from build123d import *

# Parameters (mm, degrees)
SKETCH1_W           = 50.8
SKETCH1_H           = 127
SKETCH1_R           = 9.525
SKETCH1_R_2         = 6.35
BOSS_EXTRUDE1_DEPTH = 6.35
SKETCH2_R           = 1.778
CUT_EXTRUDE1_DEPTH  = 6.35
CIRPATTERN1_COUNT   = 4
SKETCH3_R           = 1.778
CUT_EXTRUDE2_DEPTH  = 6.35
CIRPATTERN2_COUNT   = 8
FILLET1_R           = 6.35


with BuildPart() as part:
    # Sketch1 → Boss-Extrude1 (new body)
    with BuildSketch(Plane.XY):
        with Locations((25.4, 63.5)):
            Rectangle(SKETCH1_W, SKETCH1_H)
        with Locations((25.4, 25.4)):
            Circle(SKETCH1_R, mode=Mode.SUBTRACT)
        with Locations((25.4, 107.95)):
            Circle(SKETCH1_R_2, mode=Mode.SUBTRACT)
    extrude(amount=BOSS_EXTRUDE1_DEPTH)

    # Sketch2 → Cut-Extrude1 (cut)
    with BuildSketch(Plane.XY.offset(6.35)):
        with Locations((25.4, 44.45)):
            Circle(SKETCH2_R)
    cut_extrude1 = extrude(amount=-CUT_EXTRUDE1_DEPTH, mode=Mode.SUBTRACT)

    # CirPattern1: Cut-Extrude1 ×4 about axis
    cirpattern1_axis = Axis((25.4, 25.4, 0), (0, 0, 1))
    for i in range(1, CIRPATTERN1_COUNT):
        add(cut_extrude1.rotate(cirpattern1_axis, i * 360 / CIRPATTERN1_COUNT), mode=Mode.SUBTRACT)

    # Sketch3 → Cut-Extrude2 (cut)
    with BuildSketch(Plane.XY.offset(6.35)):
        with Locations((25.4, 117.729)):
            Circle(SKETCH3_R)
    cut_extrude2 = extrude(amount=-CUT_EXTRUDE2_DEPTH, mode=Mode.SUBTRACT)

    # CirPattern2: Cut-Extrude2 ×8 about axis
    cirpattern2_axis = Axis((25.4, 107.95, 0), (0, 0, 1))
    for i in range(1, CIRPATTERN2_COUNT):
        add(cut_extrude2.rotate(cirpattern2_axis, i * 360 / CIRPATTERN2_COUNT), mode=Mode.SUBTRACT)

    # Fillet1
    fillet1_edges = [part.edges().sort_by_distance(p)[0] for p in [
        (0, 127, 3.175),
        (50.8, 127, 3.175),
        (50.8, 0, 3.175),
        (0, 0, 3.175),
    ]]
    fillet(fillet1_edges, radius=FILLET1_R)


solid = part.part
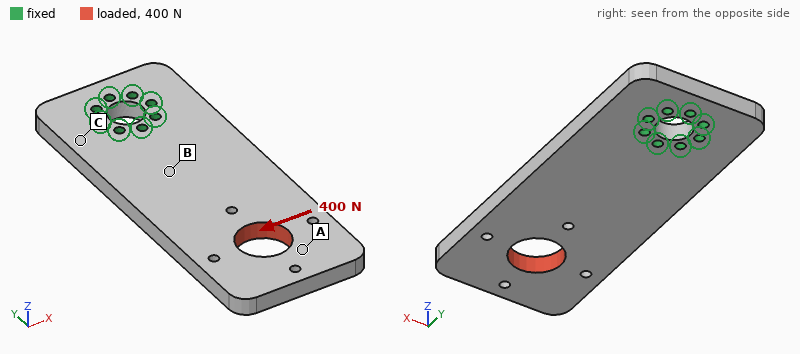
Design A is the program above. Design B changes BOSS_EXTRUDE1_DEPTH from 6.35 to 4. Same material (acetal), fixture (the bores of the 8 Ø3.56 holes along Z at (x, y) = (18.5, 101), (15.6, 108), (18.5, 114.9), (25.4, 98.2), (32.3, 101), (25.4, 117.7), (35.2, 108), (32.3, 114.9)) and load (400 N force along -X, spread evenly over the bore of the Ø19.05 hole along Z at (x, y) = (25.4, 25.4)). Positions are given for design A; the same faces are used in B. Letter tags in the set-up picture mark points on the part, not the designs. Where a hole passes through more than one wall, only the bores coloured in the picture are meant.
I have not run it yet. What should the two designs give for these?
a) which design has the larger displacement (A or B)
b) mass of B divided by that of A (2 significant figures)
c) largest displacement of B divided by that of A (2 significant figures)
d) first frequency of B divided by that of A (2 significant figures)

B
0.63
1.6
0.64
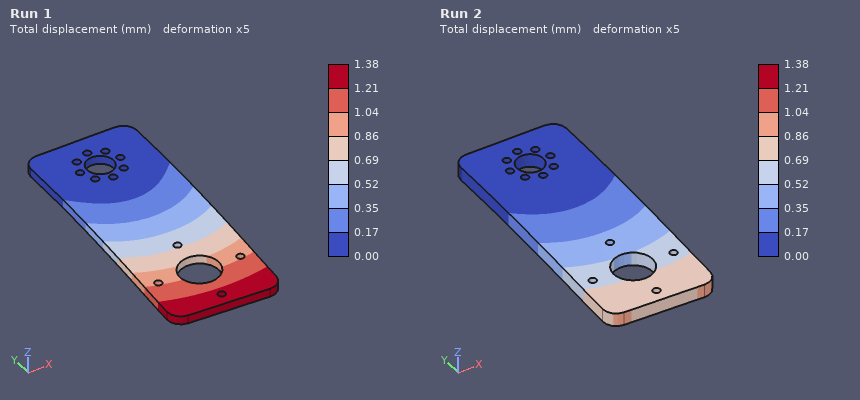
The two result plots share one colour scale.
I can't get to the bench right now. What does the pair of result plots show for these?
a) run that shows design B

Run 1
